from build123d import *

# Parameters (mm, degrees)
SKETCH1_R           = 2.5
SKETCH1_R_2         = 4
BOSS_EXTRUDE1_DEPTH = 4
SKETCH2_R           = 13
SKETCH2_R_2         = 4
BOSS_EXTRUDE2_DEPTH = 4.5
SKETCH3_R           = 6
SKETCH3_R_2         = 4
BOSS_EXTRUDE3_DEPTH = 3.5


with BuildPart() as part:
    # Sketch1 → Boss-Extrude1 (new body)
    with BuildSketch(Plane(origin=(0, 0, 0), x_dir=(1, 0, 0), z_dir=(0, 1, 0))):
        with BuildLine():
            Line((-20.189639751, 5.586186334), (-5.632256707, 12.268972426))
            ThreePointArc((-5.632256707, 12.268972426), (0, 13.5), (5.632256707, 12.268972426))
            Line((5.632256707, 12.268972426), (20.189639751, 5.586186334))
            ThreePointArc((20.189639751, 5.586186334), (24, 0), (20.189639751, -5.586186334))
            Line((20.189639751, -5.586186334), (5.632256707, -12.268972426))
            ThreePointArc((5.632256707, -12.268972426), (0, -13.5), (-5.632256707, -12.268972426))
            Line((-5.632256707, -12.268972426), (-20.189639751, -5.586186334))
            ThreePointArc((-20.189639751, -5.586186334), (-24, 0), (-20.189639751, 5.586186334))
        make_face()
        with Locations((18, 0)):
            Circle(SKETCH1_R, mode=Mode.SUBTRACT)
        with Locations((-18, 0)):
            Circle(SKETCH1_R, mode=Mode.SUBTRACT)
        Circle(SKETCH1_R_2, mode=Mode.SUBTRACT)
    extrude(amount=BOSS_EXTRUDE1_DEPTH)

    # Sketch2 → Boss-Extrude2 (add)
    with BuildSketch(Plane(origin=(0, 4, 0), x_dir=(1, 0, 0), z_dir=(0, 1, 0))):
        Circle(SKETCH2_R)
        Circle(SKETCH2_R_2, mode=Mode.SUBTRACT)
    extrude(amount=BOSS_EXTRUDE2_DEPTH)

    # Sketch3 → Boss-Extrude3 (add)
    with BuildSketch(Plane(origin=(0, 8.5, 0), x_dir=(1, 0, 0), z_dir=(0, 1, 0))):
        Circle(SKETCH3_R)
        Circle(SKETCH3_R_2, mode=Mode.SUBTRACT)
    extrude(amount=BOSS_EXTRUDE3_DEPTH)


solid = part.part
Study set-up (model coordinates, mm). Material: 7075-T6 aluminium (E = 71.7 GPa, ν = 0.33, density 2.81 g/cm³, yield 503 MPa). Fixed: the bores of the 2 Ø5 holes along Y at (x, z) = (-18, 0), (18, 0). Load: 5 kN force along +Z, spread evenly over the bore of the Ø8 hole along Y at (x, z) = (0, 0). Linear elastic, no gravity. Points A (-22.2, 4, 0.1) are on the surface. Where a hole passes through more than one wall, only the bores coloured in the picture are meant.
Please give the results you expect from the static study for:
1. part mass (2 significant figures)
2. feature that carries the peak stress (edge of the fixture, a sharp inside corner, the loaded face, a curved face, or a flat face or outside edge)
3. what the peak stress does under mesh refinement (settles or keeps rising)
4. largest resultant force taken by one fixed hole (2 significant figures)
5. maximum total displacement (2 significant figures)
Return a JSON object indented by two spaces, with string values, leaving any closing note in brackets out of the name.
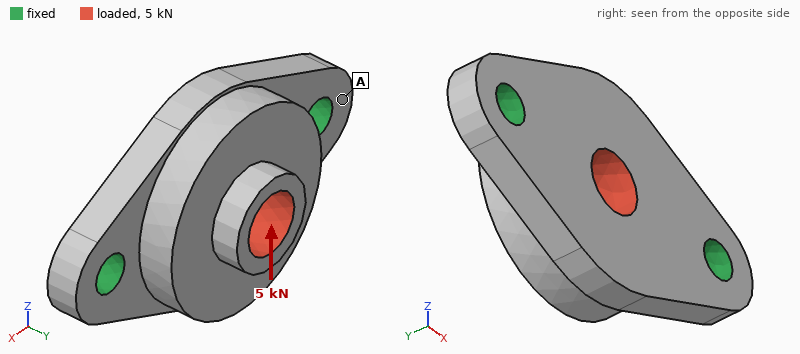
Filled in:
{
  "part mass": "16 g",
  "feature that carries the peak stress": "edge of the fixture",
  "what the peak stress does under mesh refinement": "keeps rising",
  "largest resultant force taken by one fixed hole": "2.5 kN",
  "maximum total displacement": "93 µm"
}
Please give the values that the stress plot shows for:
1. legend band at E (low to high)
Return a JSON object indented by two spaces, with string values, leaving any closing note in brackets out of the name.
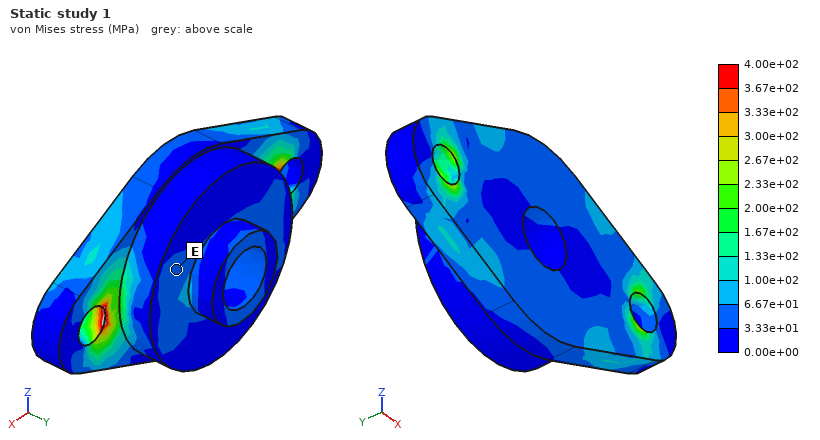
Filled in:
{
  "legend band at E": "3.33e+01 to 6.67e+01 MPa"
}
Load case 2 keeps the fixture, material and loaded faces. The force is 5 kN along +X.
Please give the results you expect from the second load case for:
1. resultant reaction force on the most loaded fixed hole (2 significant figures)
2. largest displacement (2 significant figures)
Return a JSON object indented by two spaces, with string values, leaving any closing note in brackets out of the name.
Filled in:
{
  "resultant reaction force on the most loaded fixed hole": "2.6 kN",
  "largest displacement": "16 µm"
}
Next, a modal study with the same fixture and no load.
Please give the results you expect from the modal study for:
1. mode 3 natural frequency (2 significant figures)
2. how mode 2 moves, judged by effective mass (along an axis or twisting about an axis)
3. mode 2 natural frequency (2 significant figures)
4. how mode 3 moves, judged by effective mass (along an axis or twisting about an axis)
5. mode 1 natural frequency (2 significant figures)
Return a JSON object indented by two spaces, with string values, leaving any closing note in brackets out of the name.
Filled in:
{
  "mode 3 natural frequency": "27 kHz",
  "how mode 2 moves, judged by effective mass": "along Y",
  "mode 2 natural frequency": "16 kHz",
  "how mode 3 moves, judged by effective mass": "along Z",
  "mode 1 natural frequency": "11 kHz"
}
